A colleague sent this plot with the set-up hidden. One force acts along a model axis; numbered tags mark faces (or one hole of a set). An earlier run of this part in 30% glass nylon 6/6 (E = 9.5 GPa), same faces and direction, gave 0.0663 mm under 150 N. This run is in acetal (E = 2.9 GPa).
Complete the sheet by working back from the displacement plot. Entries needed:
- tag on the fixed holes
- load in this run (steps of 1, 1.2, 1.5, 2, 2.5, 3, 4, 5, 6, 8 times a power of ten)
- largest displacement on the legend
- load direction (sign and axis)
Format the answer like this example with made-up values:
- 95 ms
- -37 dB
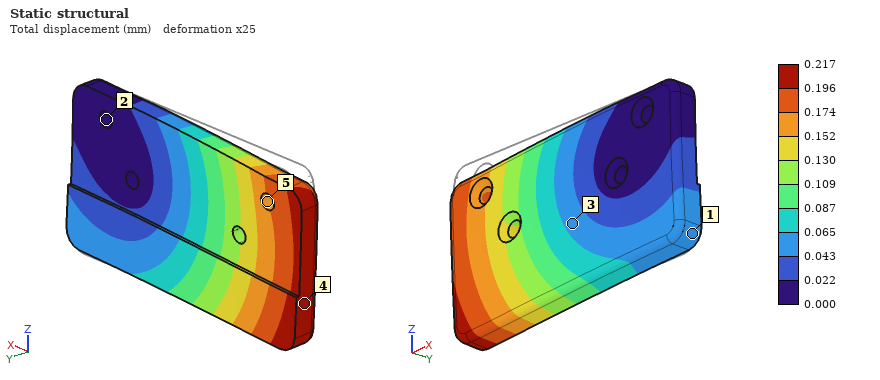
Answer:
- 2
- 150 N
- 0.217 mm
- -Z
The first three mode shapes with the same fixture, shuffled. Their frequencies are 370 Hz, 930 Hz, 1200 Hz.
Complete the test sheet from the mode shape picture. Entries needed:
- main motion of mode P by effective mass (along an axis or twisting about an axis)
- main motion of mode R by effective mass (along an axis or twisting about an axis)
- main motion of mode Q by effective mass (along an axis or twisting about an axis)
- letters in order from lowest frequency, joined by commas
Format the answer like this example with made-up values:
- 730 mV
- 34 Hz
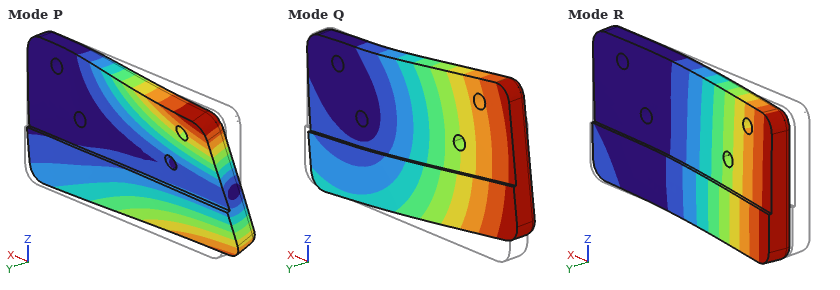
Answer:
- twisting about X
- along Y
- along Z
- R, P, Q
